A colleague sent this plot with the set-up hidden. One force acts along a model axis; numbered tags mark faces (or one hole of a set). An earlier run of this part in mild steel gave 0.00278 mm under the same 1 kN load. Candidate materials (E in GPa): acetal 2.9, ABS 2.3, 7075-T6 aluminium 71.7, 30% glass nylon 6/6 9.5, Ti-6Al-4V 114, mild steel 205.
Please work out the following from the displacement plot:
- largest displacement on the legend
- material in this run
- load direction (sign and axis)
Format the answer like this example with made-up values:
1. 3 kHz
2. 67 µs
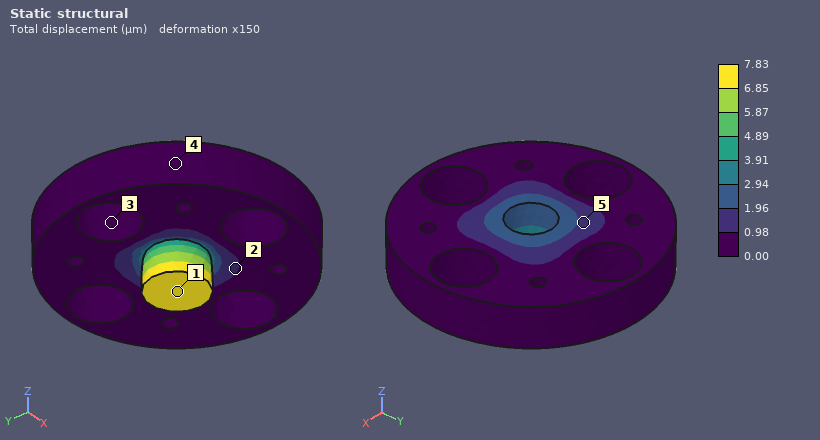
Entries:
1. 7.83 µm
2. 7075-T6 aluminium
3. +Z
